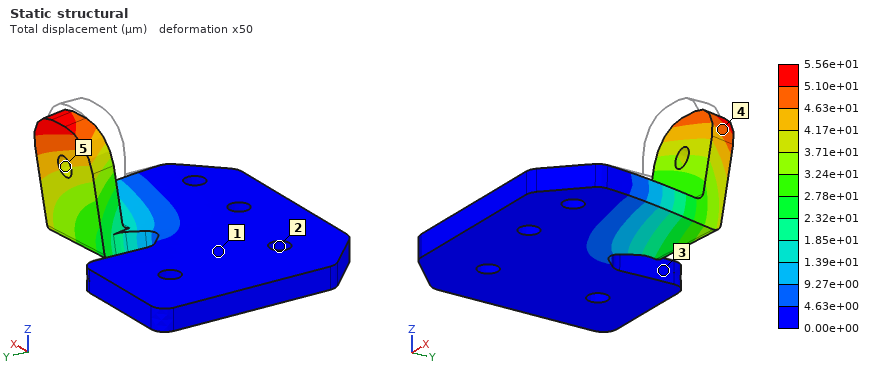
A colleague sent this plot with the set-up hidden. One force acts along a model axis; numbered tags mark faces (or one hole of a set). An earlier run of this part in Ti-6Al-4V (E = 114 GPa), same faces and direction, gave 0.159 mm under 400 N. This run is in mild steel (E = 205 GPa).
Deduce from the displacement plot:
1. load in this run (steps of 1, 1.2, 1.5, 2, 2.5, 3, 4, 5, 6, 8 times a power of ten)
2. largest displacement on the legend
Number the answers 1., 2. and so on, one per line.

1. 250 N
2. 5.56e+01 µm
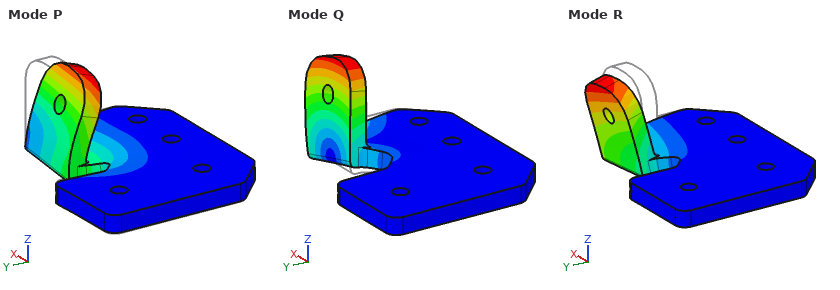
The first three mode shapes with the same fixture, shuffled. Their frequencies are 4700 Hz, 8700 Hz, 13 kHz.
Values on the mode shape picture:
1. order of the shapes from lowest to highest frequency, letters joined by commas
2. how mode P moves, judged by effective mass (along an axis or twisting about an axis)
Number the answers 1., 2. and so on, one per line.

1. R, Q, P
2. along Z
